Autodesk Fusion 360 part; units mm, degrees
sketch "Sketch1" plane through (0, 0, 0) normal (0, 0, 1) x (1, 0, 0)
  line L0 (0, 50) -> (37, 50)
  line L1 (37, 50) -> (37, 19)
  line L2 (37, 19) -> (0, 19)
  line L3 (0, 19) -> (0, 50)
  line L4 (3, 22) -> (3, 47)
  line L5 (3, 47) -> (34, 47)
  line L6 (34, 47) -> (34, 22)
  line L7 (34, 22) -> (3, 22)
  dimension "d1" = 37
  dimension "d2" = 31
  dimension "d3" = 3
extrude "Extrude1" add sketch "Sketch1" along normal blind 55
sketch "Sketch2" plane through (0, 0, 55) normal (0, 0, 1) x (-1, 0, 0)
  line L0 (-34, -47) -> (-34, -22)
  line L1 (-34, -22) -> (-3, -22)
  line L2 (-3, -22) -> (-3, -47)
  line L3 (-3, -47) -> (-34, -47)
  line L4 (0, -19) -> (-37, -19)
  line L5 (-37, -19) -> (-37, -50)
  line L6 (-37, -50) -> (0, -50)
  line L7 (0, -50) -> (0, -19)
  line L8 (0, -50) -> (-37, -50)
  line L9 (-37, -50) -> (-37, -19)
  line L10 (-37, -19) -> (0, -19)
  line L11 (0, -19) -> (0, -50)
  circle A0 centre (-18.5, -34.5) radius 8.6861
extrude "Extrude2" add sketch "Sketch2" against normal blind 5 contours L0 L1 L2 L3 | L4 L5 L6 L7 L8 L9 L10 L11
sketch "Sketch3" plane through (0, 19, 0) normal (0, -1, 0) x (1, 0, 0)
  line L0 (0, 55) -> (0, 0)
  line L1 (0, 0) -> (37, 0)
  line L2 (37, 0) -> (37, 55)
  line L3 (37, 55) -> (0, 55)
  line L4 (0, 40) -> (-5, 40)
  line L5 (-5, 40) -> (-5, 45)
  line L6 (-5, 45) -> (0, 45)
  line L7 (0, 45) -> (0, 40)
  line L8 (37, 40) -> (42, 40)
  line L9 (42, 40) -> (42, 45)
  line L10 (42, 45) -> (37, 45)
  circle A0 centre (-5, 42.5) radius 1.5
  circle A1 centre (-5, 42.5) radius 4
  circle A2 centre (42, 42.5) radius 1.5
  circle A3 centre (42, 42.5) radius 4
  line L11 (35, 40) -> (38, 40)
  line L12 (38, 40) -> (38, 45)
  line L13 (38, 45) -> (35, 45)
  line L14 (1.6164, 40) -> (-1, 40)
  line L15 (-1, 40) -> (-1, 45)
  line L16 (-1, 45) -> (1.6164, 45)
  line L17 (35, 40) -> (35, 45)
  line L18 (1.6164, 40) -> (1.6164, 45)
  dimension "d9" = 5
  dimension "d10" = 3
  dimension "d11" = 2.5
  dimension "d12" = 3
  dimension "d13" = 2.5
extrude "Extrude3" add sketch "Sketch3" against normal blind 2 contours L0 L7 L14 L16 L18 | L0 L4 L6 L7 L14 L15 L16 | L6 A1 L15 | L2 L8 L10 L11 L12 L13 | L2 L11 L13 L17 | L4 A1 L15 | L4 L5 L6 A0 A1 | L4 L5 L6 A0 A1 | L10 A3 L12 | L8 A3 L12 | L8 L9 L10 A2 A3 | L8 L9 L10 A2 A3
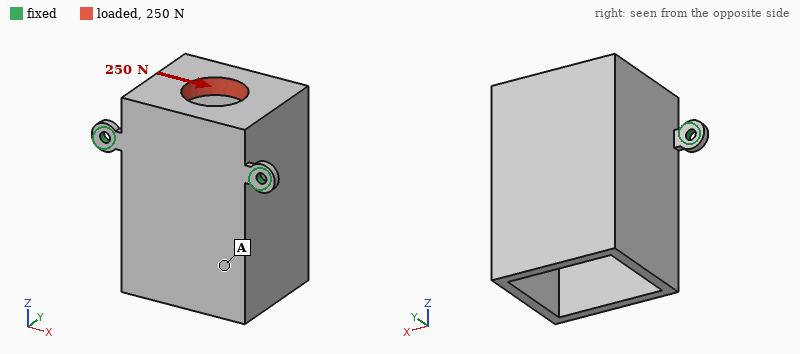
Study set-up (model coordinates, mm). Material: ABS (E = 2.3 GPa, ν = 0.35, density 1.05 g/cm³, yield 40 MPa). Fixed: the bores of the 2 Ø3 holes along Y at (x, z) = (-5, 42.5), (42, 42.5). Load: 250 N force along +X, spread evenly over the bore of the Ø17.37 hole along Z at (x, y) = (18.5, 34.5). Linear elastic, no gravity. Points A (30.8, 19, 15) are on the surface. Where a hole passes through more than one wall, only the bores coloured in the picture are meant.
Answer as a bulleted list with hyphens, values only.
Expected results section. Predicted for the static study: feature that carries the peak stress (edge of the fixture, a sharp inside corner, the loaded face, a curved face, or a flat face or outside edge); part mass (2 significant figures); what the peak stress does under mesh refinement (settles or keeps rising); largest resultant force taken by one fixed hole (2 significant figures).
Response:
- edge of the fixture
- 25 g
- keeps rising
- 170 N
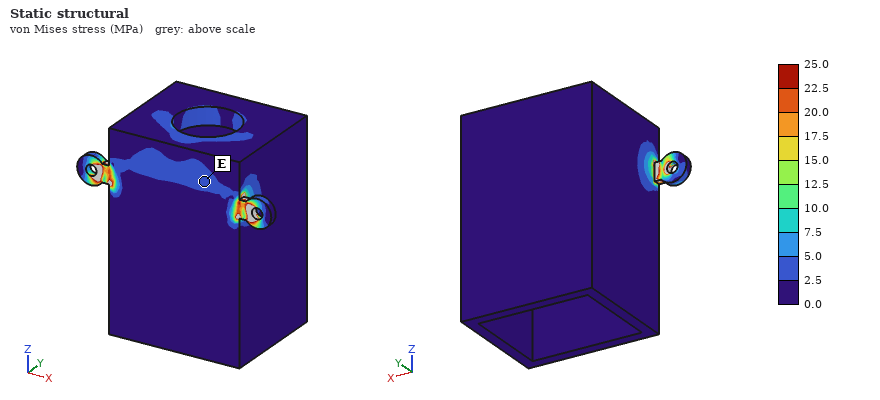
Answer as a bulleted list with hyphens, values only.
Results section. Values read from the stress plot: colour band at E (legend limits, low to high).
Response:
- 2.5 to 5.0 MPa
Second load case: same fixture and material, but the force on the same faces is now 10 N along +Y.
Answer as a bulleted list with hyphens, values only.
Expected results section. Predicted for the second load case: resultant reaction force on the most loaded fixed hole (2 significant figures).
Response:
- 5.4 N
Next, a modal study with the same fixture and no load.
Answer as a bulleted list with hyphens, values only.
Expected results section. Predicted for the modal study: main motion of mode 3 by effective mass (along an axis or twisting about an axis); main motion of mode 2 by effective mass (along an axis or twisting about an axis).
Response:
- along Y
- along X
